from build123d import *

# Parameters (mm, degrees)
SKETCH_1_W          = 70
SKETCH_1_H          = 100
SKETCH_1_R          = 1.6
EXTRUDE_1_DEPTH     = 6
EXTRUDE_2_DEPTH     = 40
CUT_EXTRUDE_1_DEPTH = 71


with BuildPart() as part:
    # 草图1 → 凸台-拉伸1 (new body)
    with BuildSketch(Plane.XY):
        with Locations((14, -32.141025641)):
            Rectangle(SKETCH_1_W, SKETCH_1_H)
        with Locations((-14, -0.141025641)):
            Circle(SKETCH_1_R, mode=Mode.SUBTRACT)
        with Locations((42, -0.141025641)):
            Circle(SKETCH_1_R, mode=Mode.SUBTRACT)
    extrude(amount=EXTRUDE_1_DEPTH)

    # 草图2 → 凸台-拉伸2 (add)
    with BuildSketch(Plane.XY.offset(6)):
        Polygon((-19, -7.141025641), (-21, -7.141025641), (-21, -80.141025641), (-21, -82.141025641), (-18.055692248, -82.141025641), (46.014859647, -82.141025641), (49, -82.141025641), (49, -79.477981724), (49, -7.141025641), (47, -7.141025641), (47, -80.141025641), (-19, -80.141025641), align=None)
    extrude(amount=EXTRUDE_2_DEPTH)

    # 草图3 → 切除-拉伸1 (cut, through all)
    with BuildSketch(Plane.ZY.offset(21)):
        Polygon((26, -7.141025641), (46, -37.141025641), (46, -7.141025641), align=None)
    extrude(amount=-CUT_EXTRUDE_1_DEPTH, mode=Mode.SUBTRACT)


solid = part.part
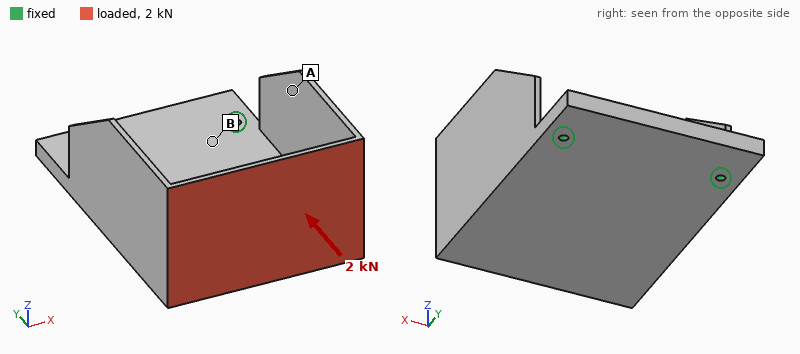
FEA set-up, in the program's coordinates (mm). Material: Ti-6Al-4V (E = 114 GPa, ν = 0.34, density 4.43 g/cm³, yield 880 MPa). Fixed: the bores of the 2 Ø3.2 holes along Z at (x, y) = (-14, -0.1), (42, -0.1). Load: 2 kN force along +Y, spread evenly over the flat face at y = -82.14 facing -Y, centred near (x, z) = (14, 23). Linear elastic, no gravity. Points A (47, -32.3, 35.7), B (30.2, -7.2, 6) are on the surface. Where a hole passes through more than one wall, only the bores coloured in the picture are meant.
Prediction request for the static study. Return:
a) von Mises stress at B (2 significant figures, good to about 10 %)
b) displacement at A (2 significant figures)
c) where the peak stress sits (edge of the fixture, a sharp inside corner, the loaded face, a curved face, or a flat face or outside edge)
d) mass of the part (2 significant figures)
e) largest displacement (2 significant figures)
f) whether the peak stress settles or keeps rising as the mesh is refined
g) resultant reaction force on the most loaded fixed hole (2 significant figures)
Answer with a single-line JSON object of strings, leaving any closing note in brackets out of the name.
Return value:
{"von Mises stress at B": "65 MPa", "displacement at A": "0.31 mm", "where the peak stress sits": "edge of the fixture", "mass of the part": "260 g", "largest displacement": "1.0 mm", "whether the peak stress settles or keeps rising as the mesh is refined": "keeps rising", "resultant reaction force on the most loaded fixed hole": "1.0 kN"}
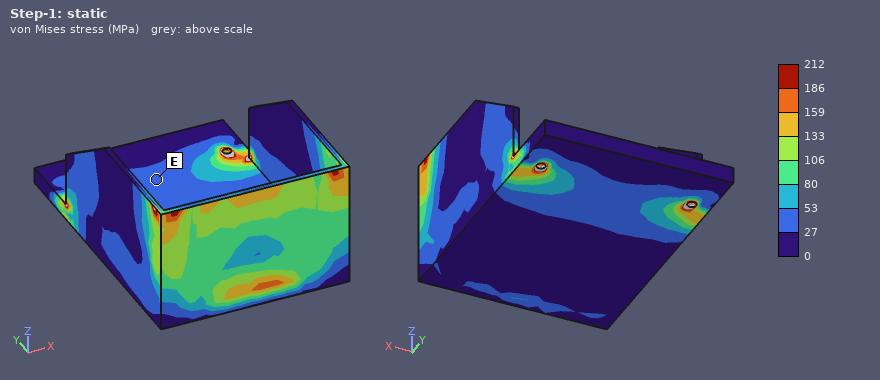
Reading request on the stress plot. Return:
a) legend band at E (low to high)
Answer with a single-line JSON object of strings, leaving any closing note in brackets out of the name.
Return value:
{"legend band at E": "27 to 53 MPa"}
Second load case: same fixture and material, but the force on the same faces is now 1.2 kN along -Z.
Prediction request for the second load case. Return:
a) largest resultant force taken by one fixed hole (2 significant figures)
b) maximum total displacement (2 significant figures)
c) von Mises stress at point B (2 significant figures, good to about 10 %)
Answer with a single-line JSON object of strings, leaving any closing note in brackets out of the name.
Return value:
{"largest resultant force taken by one fixed hole": "650 N", "maximum total displacement": "1.4 mm", "von Mises stress at point B": "140 MPa"}
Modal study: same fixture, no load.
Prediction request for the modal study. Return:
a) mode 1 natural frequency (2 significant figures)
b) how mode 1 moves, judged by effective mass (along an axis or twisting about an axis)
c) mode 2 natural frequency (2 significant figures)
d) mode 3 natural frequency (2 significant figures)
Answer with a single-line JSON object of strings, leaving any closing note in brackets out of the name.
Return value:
{"mode 1 natural frequency": "520 Hz", "how mode 1 moves, judged by effective mass": "along Z", "mode 2 natural frequency": "980 Hz", "mode 3 natural frequency": "1600 Hz"}
